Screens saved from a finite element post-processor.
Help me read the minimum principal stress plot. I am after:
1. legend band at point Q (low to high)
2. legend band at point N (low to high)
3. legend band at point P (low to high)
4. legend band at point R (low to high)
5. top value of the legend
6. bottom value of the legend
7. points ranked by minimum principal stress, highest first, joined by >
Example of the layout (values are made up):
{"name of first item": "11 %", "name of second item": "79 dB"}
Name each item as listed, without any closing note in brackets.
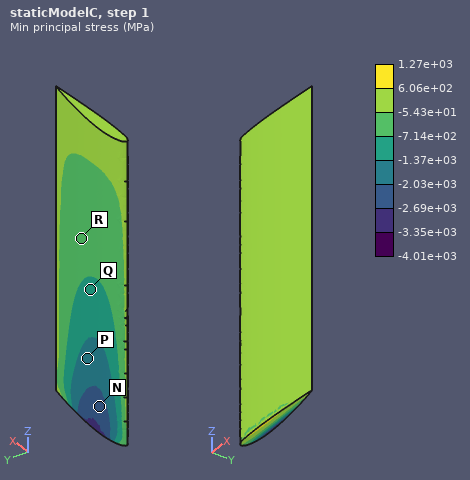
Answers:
{"legend band at point Q": "-1.37e+03 to -7.14e+02 MPa", "legend band at point N": "-2.69e+03 to -2.03e+03 MPa", "legend band at point P": "-2.03e+03 to -1.37e+03 MPa", "legend band at point R": "-7.14e+02 to -5.43e+01 MPa", "top value of the legend": "1.27e+03 MPa", "bottom value of the legend": "-4.01e+03 MPa", "points ranked by minimum principal stress, highest first, joined by >": "R > Q > P > N"}
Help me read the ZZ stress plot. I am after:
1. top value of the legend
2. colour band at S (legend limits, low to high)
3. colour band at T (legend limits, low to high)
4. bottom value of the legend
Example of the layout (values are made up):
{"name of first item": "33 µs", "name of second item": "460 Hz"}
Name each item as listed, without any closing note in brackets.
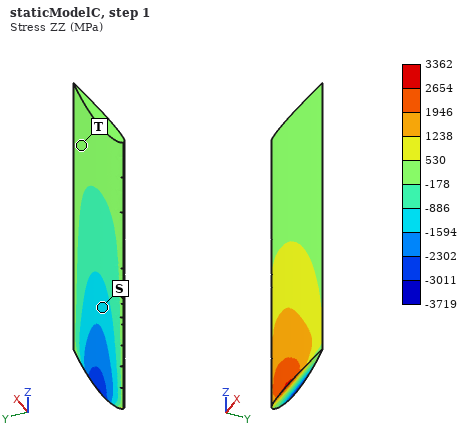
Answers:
{"top value of the legend": "3362 MPa", "colour band at S": "-1594 to -886 MPa", "colour band at T": "-178 to 530 MPa", "bottom value of the legend": "-3719 MPa"}
